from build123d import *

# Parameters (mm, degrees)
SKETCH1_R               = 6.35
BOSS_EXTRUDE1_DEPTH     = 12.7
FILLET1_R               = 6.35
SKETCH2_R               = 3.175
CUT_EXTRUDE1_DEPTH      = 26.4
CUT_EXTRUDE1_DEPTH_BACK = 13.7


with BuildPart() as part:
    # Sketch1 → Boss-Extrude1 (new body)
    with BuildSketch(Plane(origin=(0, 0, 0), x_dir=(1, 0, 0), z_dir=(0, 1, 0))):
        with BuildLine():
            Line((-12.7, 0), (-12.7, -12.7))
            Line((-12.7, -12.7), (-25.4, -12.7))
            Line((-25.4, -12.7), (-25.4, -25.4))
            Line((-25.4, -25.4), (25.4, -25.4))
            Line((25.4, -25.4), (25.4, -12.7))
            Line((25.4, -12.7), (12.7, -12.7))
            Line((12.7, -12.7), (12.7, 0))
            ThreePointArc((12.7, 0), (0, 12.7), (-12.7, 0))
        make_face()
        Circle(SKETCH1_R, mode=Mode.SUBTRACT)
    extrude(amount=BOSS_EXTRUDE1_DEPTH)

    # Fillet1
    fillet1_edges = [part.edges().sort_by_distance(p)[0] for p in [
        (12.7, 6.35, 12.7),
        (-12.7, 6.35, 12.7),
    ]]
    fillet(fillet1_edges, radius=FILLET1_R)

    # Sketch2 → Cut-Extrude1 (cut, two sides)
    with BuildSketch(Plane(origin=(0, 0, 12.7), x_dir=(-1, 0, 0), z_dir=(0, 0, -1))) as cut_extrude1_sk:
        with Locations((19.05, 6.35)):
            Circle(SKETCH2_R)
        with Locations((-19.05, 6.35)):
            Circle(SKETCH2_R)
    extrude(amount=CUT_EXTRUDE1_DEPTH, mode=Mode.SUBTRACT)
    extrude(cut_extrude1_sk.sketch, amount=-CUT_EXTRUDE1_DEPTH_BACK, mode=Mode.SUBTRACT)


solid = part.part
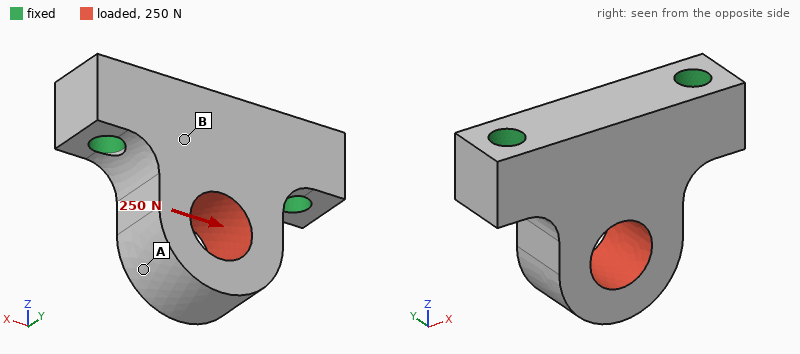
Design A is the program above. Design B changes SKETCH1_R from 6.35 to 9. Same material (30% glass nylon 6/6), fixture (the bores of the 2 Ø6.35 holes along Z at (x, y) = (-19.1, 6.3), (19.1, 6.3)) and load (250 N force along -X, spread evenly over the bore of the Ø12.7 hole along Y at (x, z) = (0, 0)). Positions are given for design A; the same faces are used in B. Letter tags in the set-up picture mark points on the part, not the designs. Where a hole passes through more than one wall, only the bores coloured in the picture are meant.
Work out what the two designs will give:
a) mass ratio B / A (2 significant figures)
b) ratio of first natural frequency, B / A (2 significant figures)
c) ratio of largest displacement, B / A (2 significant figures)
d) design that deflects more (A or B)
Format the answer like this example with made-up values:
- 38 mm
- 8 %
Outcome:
- 0.88
- 1.1
- 3.0
- B
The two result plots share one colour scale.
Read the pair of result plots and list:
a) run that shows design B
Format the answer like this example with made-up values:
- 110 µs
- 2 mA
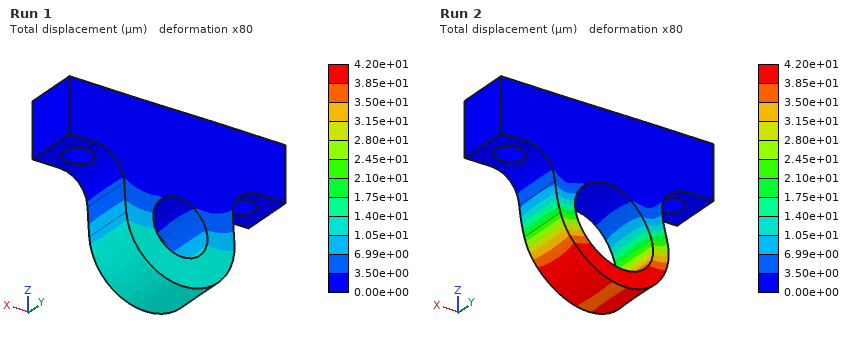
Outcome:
- Run 2
